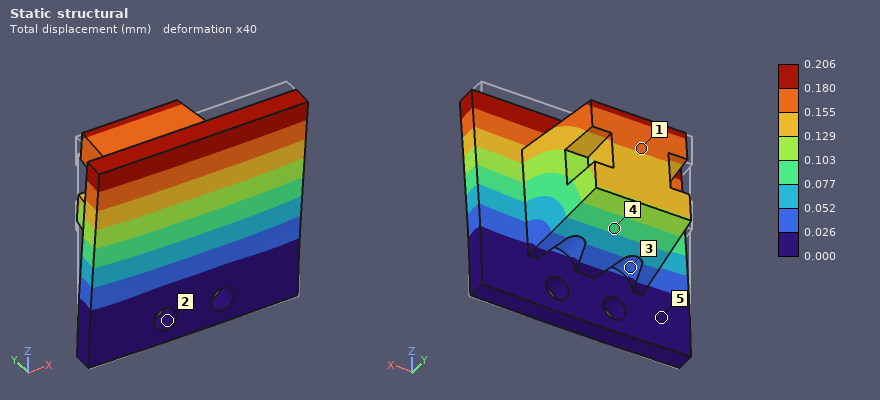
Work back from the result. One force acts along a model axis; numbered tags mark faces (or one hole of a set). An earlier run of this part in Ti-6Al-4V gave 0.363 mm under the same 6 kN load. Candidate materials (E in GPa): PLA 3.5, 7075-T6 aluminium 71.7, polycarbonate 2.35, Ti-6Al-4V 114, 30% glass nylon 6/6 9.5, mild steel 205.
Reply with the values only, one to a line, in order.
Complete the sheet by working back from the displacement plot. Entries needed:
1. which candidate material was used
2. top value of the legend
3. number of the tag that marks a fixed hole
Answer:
mild steel
0.206 mm
2
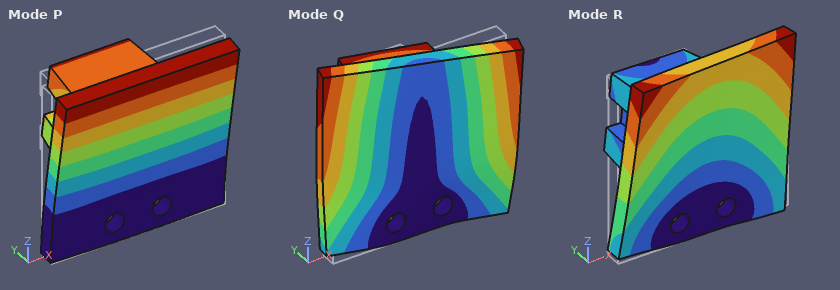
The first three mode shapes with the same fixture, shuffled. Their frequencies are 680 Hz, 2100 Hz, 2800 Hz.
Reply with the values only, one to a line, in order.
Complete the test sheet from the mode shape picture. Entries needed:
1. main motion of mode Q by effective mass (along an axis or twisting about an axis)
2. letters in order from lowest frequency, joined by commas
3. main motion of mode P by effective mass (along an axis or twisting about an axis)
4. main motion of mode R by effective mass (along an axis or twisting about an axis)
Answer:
along X
P, Q, R
along Y
along X
